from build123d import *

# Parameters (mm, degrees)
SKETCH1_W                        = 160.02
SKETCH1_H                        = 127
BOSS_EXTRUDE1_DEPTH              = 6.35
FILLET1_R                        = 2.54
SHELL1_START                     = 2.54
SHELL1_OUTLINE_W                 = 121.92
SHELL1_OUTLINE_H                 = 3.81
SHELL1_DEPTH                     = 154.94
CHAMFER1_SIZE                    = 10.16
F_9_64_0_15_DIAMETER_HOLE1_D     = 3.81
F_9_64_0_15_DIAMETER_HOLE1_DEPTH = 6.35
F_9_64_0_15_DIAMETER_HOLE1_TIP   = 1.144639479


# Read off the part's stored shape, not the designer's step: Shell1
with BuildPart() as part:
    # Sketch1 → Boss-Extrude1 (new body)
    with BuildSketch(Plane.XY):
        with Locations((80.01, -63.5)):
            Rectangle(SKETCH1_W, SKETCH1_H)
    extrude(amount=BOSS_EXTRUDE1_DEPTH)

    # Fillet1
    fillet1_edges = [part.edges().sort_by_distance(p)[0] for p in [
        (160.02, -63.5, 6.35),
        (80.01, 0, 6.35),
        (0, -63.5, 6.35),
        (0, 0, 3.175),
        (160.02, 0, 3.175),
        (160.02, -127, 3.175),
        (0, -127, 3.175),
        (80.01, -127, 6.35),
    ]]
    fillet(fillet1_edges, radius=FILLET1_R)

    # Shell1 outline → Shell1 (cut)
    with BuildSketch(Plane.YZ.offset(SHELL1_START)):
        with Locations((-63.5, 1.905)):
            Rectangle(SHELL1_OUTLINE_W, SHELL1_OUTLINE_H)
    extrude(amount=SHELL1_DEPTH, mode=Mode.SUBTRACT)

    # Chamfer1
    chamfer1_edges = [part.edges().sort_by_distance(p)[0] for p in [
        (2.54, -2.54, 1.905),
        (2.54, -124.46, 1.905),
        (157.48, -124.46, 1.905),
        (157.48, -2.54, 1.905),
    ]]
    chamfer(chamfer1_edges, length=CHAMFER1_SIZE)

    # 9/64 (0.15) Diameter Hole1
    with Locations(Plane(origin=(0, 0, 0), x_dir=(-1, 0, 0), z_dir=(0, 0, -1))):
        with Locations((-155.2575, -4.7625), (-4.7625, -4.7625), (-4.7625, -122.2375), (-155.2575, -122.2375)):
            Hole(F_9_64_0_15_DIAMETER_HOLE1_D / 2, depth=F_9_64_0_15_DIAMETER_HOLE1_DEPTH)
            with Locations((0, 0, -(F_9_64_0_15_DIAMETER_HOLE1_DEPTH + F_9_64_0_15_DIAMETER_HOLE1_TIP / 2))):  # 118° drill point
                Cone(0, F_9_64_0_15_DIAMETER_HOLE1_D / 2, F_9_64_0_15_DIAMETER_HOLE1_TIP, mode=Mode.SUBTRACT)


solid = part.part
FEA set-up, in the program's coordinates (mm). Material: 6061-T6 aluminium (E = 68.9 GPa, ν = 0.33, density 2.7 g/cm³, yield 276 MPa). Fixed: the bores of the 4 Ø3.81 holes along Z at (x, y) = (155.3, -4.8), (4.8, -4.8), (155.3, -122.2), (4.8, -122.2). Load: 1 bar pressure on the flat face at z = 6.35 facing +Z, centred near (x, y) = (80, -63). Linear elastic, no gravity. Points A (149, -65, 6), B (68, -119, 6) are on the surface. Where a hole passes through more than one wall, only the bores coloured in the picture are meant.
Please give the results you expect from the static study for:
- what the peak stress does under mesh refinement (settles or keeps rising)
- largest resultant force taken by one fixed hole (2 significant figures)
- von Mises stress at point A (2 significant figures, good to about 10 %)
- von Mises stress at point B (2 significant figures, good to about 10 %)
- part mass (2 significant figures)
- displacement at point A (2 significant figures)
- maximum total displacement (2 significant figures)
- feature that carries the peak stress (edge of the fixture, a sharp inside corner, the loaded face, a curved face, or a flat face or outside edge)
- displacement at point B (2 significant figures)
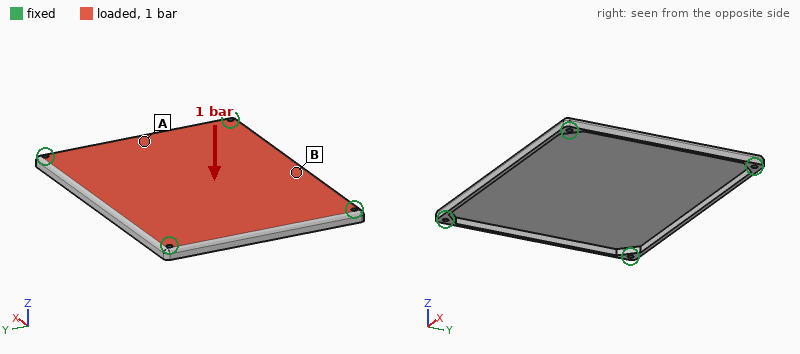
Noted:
keeps rising
830 N
39 MPa
56 MPa
150 g
0.46 mm
1.6 mm
edge of the fixture
0.79 mm
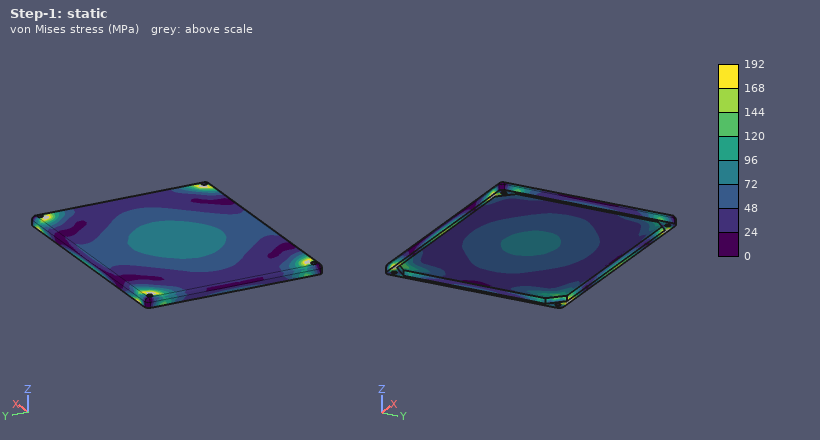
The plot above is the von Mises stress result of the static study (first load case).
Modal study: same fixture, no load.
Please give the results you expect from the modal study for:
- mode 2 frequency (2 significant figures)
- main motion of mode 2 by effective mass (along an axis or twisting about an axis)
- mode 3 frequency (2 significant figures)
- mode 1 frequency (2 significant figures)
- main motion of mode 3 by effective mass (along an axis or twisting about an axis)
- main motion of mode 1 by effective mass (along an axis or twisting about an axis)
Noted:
1100 Hz
twisting about X
1300 Hz
580 Hz
twisting about Y
along Z
